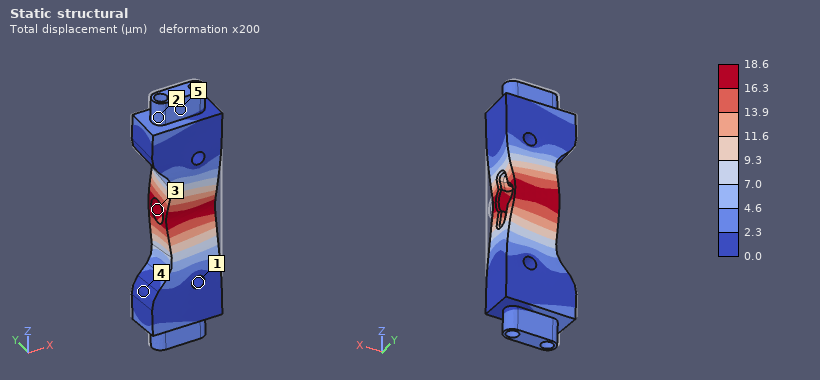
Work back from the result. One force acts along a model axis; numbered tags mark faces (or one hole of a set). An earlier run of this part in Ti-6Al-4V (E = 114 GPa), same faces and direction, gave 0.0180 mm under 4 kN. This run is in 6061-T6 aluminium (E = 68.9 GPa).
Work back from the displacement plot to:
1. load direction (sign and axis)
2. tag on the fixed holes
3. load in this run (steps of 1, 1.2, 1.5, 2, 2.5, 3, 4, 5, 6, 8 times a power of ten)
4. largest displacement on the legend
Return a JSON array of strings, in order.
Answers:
["+Y", "1", "2.5 kN", "18.6 µm"]
